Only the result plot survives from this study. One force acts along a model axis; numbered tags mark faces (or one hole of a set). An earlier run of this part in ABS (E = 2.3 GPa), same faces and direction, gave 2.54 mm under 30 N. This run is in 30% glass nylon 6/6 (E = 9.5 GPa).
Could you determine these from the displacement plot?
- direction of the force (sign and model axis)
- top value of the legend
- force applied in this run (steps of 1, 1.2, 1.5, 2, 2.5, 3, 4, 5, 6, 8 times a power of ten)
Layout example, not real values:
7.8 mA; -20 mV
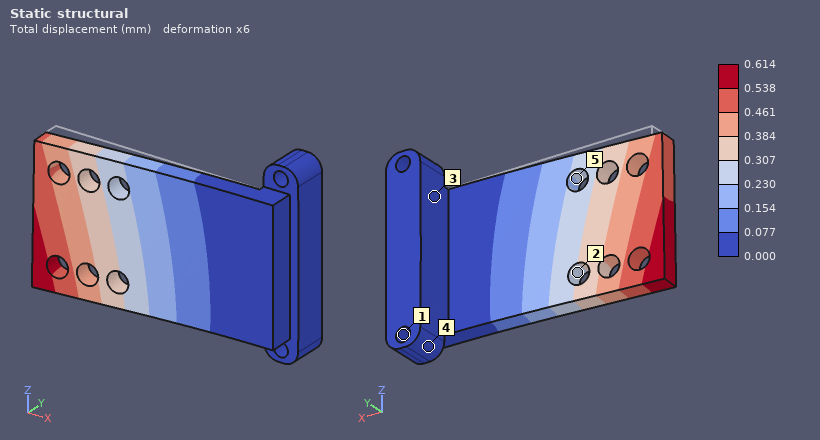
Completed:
-Y; 0.614 mm; 30 N
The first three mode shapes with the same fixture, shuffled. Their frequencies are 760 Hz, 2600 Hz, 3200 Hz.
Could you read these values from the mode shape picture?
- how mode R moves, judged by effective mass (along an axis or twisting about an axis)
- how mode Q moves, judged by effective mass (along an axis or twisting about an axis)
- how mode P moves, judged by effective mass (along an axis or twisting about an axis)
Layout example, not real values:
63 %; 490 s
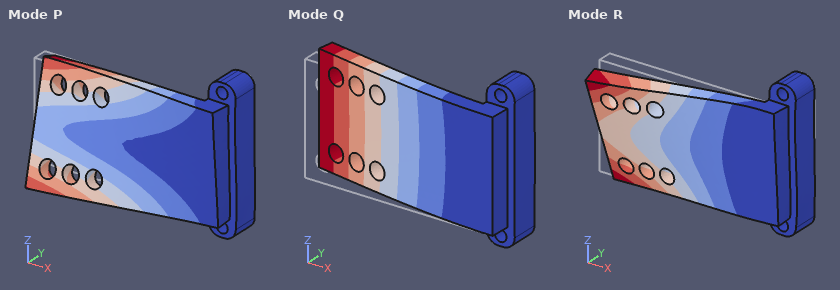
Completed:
along Z; along Y; along Z
